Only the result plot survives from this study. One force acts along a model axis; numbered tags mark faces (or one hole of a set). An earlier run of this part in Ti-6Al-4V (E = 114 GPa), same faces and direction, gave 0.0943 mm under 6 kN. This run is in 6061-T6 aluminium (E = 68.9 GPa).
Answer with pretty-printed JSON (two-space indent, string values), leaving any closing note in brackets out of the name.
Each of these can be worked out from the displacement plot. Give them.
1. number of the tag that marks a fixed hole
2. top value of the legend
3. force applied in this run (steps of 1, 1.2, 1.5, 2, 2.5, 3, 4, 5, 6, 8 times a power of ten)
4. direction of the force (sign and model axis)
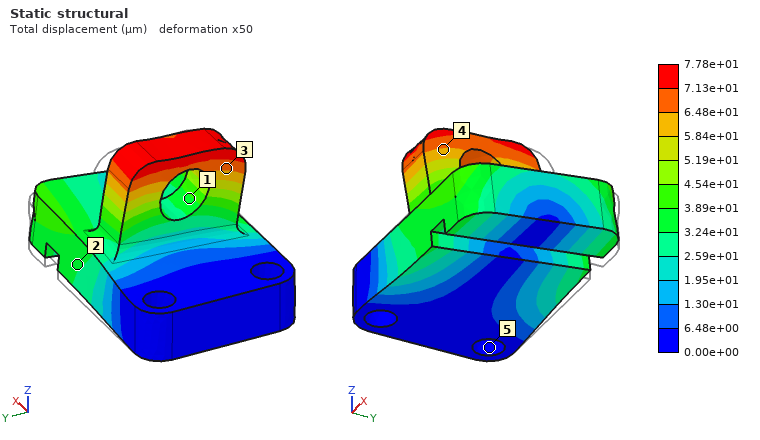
{
  "number of the tag that marks a fixed hole": "5",
  "top value of the legend": "7.78e+01 µm",
  "force applied in this run": "3 kN",
  "direction of the force": "-Y"
}
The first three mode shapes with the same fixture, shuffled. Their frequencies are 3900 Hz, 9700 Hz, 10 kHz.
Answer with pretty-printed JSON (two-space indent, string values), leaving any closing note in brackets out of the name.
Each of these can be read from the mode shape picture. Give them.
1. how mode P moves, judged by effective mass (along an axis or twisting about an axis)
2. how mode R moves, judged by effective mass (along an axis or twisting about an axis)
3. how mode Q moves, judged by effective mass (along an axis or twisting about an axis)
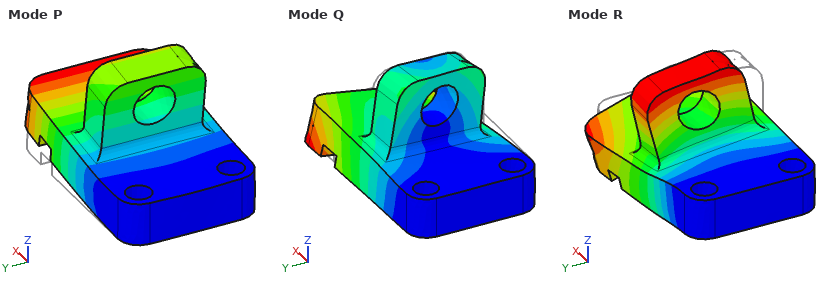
{
  "how mode P moves, judged by effective mass": "along Z",
  "how mode R moves, judged by effective mass": "along Y",
  "how mode Q moves, judged by effective mass": "along Y"
}
